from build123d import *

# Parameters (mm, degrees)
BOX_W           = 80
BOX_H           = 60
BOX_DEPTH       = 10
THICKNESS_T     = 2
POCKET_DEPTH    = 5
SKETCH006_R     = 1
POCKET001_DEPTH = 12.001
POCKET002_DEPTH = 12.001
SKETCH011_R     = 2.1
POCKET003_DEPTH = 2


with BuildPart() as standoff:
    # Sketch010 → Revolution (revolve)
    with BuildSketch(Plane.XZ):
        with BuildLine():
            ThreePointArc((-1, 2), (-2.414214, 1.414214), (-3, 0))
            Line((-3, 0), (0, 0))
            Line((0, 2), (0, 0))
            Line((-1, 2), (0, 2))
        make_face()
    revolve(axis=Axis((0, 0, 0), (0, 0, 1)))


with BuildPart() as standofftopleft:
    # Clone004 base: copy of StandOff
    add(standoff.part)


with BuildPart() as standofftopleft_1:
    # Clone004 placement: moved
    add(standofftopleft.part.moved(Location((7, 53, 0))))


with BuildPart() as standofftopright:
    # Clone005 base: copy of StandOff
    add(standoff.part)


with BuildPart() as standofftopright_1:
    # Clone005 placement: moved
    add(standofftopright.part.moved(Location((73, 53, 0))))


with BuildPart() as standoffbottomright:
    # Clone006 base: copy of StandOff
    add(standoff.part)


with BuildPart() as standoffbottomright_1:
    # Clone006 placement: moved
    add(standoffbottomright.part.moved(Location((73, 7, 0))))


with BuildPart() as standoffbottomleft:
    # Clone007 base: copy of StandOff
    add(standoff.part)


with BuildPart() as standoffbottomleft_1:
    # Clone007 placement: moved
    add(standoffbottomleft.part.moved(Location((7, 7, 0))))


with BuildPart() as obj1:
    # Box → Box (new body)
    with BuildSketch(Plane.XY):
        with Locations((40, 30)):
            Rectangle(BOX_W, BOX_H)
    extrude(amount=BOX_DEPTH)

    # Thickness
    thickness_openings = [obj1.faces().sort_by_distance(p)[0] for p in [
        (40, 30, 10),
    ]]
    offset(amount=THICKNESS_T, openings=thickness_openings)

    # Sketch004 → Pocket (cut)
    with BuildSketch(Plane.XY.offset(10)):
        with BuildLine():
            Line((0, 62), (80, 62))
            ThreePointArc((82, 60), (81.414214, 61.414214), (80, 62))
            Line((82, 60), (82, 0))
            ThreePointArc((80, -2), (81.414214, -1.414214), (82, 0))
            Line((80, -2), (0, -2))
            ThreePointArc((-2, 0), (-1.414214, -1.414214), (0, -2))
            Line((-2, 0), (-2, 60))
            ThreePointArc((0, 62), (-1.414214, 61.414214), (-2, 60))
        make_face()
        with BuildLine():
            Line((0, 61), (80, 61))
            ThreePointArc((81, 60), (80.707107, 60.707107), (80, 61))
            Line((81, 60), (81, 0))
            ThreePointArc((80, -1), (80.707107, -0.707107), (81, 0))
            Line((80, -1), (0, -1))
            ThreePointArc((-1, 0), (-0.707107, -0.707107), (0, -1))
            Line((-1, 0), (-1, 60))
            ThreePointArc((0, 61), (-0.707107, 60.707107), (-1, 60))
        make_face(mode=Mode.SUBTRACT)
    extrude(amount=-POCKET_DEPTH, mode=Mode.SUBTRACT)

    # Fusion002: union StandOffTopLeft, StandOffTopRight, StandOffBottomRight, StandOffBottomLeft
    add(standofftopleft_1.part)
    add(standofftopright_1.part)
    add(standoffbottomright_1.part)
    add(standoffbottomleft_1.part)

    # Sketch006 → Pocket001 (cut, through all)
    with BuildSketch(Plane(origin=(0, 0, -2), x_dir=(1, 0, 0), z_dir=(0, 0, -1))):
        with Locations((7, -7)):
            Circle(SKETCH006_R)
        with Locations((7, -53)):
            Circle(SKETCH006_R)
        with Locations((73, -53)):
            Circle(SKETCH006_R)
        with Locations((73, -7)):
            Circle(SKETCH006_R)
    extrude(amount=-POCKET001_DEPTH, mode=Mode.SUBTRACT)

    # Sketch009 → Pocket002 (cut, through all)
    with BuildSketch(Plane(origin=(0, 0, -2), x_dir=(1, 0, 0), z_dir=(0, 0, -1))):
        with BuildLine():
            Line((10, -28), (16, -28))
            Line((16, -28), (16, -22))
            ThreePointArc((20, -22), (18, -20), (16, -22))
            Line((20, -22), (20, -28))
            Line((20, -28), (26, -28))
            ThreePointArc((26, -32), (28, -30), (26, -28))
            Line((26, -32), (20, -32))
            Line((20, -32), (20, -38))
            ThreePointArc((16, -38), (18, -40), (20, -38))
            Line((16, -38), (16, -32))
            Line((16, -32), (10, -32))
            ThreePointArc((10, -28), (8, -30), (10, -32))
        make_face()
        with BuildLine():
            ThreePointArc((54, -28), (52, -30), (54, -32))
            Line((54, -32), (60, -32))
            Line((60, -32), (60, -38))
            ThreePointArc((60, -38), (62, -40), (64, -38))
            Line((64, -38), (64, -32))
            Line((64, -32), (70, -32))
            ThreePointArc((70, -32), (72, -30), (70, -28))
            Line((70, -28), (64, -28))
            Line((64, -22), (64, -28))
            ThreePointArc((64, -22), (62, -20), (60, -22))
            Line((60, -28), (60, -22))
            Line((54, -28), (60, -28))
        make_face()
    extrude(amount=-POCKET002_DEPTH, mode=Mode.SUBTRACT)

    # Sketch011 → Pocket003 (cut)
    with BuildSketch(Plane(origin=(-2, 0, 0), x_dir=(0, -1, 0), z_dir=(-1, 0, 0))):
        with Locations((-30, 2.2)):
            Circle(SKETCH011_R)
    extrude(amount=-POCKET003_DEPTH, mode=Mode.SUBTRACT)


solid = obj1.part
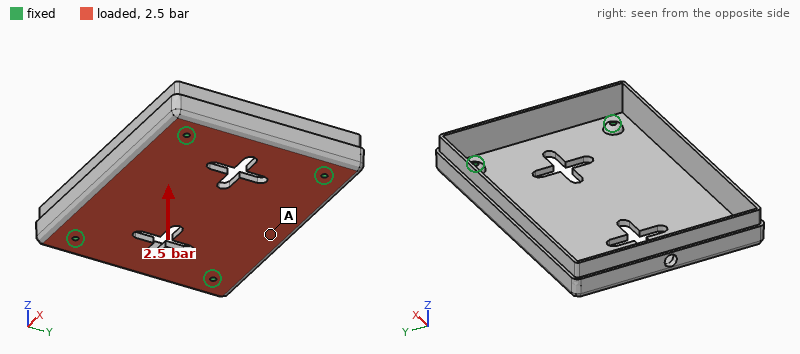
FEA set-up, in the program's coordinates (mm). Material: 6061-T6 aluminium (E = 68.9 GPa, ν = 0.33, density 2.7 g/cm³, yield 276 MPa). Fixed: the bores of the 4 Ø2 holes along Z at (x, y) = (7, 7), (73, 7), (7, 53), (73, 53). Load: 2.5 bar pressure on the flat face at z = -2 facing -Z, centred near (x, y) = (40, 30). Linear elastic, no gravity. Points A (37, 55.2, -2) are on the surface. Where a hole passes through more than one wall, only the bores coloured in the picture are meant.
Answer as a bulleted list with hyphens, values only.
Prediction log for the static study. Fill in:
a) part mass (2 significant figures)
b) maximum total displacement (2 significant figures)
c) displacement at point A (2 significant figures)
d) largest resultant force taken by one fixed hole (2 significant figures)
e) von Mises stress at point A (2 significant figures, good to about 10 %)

- 39 g
- 0.26 mm
- 0.088 mm
- 290 N
- 21 MPa
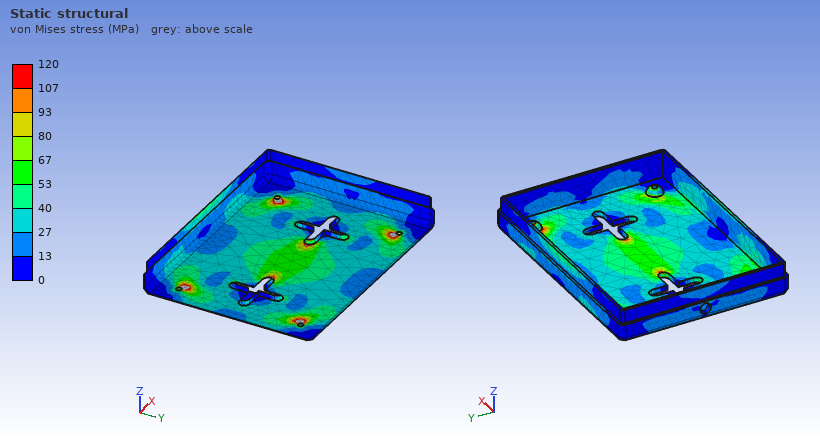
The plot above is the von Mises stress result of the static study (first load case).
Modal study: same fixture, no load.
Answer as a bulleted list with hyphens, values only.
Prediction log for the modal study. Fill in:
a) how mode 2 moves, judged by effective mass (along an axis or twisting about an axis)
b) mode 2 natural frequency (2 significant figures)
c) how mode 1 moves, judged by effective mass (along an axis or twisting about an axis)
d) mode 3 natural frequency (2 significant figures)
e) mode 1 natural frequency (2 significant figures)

- twisting about X
- 5000 Hz
- along Z
- 5200 Hz
- 2600 Hz
